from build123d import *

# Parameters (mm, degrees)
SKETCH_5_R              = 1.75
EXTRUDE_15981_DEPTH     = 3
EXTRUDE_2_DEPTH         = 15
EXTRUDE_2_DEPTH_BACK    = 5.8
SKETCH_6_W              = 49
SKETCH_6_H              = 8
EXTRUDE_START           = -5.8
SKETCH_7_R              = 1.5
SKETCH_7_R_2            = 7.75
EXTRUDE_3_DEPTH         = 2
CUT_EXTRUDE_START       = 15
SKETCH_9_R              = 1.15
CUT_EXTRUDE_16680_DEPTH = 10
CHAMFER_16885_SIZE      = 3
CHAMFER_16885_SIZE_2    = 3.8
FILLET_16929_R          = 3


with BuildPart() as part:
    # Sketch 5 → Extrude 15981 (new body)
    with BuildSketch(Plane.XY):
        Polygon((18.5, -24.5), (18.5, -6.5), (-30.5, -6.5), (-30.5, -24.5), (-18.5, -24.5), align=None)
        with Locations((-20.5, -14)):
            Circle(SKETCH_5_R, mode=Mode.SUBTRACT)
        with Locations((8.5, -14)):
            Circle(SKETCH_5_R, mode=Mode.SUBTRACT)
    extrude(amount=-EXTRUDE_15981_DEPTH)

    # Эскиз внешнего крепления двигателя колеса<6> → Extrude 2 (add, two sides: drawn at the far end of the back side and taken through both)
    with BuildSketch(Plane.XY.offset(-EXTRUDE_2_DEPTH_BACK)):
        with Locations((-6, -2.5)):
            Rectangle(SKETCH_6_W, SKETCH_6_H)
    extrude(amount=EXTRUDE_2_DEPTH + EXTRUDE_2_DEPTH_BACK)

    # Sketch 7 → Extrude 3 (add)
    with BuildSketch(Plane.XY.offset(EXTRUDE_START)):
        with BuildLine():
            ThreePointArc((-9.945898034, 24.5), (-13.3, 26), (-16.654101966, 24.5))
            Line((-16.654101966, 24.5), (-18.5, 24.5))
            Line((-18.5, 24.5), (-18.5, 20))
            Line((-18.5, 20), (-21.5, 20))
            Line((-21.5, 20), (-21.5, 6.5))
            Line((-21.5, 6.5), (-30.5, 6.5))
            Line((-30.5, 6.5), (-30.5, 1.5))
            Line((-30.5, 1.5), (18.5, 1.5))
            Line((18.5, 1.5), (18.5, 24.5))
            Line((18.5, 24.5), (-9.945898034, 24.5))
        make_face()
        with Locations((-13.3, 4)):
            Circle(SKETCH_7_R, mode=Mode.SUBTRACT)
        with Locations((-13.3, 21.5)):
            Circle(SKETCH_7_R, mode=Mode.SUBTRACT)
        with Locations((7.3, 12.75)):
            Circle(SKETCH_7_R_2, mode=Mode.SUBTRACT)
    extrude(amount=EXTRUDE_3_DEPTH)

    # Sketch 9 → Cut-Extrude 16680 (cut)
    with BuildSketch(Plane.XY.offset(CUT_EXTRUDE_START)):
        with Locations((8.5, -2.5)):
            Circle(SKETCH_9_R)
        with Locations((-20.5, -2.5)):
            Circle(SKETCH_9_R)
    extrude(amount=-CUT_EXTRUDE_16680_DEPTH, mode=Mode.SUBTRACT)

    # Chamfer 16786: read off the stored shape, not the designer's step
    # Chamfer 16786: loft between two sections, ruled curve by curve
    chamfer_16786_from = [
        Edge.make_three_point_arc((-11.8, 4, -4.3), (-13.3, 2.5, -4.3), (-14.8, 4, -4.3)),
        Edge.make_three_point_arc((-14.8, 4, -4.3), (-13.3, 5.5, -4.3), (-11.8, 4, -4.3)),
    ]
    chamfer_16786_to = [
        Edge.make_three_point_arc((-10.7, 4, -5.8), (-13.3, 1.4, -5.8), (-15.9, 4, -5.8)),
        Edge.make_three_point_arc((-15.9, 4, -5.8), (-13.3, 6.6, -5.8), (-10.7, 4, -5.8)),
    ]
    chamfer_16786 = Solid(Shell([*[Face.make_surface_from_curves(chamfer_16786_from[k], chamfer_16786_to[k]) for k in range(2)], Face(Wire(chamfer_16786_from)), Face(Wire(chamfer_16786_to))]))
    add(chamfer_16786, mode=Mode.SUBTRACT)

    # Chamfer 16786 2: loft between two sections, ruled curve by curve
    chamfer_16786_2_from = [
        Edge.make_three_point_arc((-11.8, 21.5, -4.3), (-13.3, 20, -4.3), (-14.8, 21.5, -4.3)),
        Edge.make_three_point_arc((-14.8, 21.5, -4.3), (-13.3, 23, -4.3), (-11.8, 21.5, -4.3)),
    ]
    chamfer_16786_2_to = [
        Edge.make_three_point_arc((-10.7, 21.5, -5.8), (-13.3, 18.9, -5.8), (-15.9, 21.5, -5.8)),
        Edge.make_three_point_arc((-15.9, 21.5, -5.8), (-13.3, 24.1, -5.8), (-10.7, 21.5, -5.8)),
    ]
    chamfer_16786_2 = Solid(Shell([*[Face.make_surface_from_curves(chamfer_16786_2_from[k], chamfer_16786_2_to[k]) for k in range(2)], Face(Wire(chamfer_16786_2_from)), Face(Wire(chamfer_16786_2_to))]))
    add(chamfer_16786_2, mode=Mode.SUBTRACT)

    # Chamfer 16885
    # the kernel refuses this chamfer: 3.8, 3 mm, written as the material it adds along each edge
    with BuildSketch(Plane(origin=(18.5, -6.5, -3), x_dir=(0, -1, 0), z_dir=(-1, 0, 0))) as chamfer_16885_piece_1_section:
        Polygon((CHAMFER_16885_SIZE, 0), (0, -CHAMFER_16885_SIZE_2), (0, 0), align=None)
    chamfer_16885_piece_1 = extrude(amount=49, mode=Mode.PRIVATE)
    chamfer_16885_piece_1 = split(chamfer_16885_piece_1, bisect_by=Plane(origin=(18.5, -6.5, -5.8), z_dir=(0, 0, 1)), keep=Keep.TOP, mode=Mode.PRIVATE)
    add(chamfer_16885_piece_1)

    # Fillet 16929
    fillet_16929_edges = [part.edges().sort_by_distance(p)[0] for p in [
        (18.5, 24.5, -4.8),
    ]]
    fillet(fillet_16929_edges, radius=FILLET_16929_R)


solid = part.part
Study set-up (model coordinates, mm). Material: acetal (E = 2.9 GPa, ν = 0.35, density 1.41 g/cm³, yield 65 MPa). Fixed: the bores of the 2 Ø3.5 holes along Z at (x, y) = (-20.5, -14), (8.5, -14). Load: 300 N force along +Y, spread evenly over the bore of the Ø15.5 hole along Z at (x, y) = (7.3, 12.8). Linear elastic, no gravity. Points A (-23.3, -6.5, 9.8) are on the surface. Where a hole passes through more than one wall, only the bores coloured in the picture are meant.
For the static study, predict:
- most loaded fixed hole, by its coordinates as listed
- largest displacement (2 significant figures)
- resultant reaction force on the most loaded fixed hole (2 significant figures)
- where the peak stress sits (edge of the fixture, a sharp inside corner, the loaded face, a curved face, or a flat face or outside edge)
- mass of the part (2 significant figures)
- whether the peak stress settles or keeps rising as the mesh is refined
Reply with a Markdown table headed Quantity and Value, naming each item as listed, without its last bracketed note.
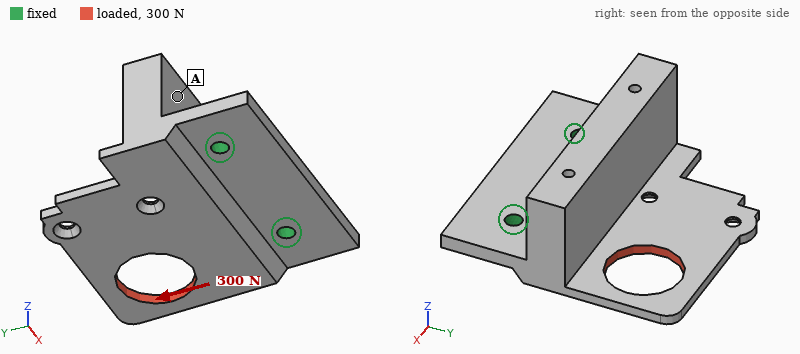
| Quantity | Value |
|---|---|
| most loaded fixed hole, by its coordinates as listed | (8.5, -14) |
| largest displacement | 0.86 mm |
| resultant reaction force on the most loaded fixed hole | 280 N |
| where the peak stress sits | edge of the fixture |
| mass of the part | 17 g |
| whether the peak stress settles or keeps rising as the mesh is refined | keeps rising |
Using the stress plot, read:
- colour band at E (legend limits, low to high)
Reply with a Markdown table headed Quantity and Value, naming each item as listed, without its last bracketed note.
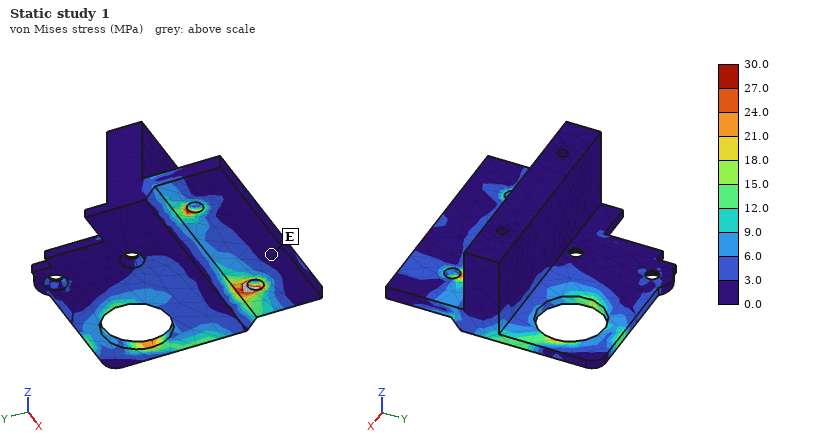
| Quantity | Value |
|---|---|
| colour band at E | 0.0 to 3.0 MPa |
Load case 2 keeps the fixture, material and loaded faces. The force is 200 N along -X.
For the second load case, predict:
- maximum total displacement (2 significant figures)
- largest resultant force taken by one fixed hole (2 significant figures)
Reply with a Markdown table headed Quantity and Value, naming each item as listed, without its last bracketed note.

| Quantity | Value |
|---|---|
| maximum total displacement | 0.19 mm |
| largest resultant force taken by one fixed hole | 200 N |
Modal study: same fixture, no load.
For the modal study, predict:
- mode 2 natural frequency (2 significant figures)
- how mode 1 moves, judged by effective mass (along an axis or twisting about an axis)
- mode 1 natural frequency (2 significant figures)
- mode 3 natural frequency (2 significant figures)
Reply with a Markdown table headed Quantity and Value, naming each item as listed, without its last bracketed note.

| Quantity | Value |
|---|---|
| mode 2 natural frequency | 1100 Hz |
| how mode 1 moves, judged by effective mass | along Z |
| mode 1 natural frequency | 540 Hz |
| mode 3 natural frequency | 1300 Hz |
